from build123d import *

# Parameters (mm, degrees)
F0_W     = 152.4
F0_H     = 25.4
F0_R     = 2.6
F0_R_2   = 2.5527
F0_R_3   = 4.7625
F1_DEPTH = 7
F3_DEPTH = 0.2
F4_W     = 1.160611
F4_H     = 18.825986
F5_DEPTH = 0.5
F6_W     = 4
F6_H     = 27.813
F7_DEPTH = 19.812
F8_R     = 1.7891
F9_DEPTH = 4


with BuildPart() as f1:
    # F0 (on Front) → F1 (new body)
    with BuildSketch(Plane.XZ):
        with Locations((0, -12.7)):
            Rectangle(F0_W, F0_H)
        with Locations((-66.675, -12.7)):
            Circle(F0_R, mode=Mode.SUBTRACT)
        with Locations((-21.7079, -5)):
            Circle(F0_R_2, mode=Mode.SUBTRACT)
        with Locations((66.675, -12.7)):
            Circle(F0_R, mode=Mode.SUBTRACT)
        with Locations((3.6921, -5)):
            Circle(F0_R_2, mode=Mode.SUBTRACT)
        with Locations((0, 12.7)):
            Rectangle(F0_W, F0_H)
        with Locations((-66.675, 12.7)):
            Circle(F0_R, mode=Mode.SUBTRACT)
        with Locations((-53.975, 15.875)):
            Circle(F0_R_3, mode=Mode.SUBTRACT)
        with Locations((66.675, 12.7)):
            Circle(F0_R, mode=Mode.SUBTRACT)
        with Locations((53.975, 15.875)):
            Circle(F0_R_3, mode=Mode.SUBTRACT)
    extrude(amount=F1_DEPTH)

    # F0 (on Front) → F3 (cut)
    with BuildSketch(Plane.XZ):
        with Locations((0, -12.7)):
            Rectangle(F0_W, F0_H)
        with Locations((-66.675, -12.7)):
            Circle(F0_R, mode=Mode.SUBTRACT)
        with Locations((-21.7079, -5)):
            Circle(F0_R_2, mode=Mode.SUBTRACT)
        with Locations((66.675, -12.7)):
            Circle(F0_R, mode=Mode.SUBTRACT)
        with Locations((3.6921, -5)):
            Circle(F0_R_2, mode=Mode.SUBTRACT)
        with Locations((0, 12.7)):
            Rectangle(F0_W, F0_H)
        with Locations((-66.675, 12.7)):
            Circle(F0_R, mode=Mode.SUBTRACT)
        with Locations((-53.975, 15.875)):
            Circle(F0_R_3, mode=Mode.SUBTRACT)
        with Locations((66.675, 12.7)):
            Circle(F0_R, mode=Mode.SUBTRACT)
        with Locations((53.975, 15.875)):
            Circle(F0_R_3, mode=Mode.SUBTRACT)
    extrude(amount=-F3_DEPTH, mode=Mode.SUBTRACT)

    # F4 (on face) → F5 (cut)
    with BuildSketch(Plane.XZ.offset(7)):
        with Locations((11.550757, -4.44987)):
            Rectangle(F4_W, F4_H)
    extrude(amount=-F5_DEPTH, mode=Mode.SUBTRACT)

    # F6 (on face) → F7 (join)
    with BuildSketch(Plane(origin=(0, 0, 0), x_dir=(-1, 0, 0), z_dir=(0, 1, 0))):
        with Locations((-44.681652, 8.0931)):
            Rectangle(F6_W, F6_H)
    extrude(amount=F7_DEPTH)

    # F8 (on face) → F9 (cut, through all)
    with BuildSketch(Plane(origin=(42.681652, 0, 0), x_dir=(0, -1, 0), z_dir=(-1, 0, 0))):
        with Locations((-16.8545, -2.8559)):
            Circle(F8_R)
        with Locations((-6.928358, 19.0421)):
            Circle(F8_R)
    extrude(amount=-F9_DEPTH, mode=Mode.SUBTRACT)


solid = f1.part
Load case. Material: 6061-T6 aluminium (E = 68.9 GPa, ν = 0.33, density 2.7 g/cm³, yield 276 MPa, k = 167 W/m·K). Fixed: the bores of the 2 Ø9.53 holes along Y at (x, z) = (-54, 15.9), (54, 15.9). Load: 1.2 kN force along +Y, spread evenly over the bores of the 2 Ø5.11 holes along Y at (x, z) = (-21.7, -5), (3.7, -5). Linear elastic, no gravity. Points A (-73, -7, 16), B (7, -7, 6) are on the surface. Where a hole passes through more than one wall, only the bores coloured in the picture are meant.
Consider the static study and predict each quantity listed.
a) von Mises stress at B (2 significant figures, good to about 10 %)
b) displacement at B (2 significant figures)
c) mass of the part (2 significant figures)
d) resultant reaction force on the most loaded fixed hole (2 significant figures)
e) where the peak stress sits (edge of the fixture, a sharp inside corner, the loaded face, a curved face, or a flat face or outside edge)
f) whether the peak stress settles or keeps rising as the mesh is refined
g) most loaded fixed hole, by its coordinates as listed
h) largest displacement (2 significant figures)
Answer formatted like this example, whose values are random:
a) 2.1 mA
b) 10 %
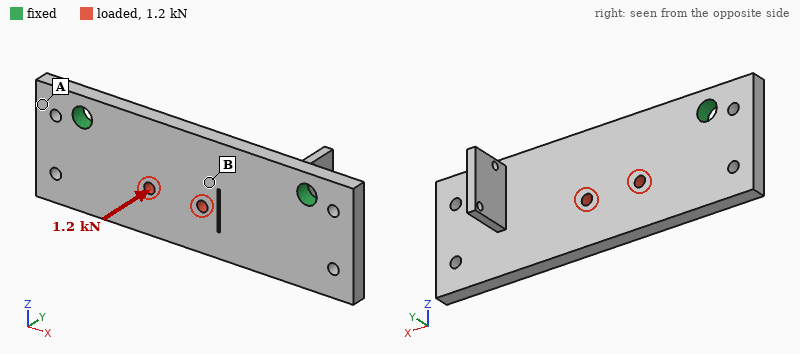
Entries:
a) 23 MPa
b) 0.078 mm
c) 150 g
d) 730 N
e) edge of the fixture
f) keeps rising
g) (-54, 15.9)
h) 0.16 mm
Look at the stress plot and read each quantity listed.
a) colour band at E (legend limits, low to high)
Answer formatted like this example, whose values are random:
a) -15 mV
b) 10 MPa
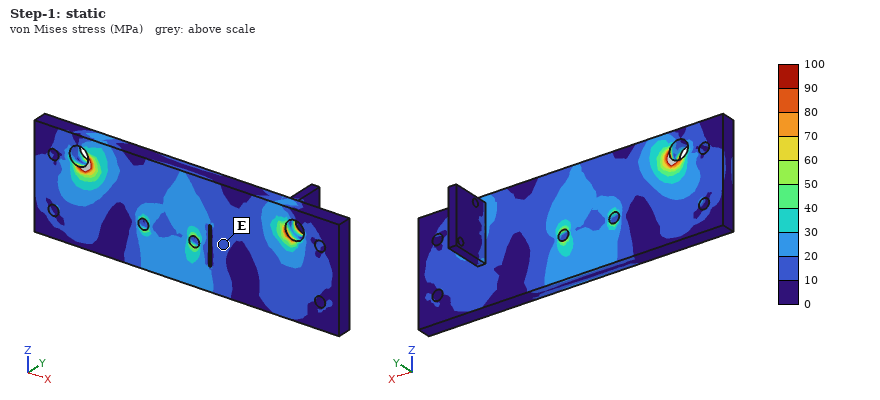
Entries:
a) 10 to 20 MPa
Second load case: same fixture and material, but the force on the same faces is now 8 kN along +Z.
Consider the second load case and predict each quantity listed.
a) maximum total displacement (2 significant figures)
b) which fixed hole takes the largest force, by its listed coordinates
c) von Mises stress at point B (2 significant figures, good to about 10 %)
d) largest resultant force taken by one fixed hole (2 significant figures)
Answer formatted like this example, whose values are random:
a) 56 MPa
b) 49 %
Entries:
a) 43 µm
b) (-54, 15.9)
c) 19 MPa
d) 5.5 kN
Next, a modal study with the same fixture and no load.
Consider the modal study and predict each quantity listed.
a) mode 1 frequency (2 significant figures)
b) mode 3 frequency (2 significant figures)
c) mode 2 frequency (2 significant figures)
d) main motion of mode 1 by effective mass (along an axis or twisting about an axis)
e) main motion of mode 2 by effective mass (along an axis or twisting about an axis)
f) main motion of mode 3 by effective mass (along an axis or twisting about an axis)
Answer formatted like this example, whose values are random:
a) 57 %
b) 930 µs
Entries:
a) 2200 Hz
b) 3900 Hz
c) 3600 Hz
d) along Y
e) twisting about X
f) twisting about Z
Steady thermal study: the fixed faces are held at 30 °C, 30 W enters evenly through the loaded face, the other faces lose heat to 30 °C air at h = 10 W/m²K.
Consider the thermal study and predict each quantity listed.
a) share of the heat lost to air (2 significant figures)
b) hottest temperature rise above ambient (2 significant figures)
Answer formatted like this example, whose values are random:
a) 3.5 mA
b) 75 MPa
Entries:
a) 4.0 %
b) 16 K
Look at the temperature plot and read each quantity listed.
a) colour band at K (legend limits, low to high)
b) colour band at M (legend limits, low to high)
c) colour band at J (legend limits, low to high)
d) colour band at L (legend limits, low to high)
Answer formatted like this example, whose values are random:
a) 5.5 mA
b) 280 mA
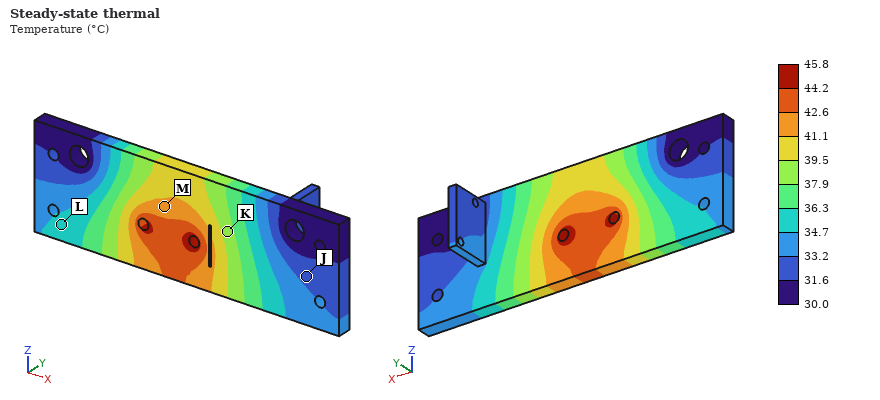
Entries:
a) 37.9 to 39.5 °C
b) 41.1 to 42.6 °C
c) 31.6 to 33.2 °C
d) 34.7 to 36.3 °C
